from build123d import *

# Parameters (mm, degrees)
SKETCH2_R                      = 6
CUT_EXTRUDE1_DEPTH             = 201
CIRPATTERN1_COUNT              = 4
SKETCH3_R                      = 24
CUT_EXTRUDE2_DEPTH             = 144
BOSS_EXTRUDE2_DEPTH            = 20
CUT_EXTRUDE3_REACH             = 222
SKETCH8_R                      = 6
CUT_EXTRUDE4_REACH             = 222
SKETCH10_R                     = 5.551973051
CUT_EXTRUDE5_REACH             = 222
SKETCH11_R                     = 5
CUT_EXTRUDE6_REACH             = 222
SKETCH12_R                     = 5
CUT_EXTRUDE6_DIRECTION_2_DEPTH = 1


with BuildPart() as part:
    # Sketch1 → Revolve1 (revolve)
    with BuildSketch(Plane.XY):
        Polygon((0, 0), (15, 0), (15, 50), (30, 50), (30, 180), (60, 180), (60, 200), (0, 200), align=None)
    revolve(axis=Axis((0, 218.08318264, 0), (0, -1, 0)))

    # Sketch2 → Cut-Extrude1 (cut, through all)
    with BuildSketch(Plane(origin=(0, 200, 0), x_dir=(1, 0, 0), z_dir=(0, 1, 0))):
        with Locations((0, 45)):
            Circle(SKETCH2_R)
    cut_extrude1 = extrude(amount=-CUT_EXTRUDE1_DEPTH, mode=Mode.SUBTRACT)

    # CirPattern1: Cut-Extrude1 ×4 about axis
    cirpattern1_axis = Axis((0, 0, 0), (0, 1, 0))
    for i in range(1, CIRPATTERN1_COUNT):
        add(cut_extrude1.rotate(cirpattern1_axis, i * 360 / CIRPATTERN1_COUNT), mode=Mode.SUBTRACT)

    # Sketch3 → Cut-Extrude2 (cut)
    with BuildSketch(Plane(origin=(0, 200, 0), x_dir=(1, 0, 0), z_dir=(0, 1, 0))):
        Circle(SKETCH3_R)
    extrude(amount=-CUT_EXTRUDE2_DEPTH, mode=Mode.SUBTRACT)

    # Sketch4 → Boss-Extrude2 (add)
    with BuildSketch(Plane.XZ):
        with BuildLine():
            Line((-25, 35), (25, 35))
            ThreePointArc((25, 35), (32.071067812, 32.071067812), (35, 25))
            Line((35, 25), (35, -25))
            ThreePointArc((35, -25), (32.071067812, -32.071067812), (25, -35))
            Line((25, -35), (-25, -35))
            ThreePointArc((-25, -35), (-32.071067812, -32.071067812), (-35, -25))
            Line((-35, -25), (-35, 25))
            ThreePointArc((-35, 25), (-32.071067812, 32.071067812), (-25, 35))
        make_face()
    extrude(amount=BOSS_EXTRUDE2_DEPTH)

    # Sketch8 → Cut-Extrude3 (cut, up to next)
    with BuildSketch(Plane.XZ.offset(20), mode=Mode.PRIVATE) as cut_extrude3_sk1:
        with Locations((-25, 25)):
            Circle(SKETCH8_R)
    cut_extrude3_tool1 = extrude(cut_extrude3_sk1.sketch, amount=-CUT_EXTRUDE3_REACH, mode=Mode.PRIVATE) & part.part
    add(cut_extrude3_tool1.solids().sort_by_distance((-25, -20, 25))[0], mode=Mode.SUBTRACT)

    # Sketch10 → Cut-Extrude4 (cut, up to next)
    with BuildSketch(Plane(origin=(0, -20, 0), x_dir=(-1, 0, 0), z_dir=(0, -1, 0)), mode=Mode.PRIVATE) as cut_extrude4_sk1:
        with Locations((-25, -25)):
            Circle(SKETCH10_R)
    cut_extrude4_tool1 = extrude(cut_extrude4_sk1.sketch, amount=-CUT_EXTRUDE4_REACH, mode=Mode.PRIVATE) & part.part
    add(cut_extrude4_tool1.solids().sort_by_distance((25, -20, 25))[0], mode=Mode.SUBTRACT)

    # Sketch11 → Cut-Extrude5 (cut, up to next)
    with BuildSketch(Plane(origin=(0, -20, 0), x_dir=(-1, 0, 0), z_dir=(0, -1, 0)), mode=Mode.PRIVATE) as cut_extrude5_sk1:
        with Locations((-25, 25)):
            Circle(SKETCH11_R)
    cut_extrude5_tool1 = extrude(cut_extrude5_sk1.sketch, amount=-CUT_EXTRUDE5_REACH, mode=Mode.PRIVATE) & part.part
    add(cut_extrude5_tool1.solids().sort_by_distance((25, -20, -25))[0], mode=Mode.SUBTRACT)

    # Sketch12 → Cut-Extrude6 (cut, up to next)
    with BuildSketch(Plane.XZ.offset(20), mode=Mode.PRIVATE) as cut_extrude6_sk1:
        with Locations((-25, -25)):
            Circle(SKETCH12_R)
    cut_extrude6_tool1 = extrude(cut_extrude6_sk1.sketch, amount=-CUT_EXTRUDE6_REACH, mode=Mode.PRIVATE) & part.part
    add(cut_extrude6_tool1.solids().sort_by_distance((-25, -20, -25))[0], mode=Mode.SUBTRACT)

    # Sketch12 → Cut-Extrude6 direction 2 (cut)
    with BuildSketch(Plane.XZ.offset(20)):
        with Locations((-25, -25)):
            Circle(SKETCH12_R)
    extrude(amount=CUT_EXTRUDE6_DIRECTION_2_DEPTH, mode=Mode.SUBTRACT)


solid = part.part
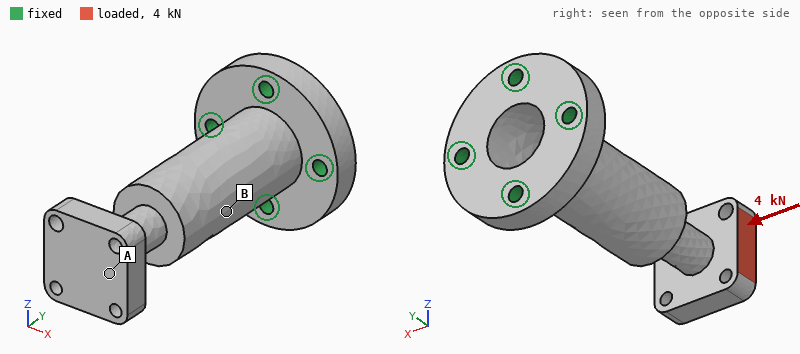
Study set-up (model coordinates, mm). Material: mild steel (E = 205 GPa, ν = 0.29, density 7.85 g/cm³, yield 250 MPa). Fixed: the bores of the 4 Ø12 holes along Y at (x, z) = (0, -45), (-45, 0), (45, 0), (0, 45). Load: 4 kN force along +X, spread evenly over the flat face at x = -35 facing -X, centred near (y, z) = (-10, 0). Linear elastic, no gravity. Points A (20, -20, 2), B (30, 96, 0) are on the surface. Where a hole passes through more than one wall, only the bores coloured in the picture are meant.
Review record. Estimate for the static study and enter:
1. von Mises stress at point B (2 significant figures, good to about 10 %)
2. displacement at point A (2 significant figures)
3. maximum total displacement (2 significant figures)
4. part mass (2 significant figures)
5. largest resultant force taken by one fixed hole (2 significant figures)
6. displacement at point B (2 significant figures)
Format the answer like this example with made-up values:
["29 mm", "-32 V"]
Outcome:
["34 MPa", "0.29 mm", "0.30 mm", "3.5 kg", "10 kN", "0.061 mm"]
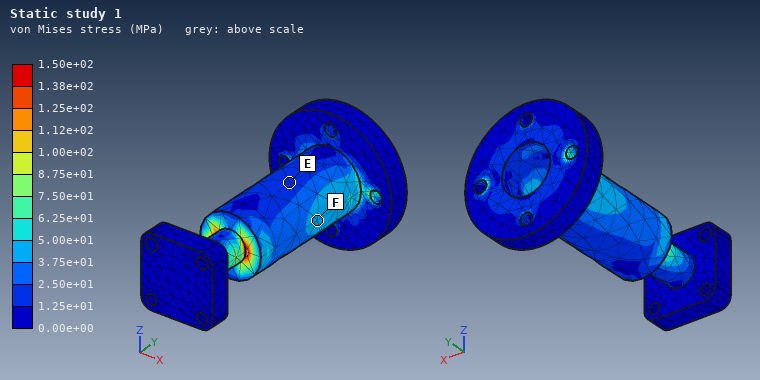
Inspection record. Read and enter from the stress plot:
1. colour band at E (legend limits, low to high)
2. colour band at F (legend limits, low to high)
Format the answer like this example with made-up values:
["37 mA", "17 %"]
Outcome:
["1.25e+01 to 2.50e+01 MPa", "3.75e+01 to 5.00e+01 MPa"]
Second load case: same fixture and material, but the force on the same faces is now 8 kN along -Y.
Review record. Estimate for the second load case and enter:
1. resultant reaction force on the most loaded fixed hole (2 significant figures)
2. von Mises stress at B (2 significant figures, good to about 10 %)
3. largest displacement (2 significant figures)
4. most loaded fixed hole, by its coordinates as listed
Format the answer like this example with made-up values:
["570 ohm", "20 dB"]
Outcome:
["5.7 kN", "15 MPa", "0.28 mm", "(-45, 0)"]
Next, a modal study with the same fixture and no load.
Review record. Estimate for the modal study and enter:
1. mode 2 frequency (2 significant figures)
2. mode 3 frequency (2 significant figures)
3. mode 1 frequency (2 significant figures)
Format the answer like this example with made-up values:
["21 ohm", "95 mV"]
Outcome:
["660 Hz", "2000 Hz", "660 Hz"]
